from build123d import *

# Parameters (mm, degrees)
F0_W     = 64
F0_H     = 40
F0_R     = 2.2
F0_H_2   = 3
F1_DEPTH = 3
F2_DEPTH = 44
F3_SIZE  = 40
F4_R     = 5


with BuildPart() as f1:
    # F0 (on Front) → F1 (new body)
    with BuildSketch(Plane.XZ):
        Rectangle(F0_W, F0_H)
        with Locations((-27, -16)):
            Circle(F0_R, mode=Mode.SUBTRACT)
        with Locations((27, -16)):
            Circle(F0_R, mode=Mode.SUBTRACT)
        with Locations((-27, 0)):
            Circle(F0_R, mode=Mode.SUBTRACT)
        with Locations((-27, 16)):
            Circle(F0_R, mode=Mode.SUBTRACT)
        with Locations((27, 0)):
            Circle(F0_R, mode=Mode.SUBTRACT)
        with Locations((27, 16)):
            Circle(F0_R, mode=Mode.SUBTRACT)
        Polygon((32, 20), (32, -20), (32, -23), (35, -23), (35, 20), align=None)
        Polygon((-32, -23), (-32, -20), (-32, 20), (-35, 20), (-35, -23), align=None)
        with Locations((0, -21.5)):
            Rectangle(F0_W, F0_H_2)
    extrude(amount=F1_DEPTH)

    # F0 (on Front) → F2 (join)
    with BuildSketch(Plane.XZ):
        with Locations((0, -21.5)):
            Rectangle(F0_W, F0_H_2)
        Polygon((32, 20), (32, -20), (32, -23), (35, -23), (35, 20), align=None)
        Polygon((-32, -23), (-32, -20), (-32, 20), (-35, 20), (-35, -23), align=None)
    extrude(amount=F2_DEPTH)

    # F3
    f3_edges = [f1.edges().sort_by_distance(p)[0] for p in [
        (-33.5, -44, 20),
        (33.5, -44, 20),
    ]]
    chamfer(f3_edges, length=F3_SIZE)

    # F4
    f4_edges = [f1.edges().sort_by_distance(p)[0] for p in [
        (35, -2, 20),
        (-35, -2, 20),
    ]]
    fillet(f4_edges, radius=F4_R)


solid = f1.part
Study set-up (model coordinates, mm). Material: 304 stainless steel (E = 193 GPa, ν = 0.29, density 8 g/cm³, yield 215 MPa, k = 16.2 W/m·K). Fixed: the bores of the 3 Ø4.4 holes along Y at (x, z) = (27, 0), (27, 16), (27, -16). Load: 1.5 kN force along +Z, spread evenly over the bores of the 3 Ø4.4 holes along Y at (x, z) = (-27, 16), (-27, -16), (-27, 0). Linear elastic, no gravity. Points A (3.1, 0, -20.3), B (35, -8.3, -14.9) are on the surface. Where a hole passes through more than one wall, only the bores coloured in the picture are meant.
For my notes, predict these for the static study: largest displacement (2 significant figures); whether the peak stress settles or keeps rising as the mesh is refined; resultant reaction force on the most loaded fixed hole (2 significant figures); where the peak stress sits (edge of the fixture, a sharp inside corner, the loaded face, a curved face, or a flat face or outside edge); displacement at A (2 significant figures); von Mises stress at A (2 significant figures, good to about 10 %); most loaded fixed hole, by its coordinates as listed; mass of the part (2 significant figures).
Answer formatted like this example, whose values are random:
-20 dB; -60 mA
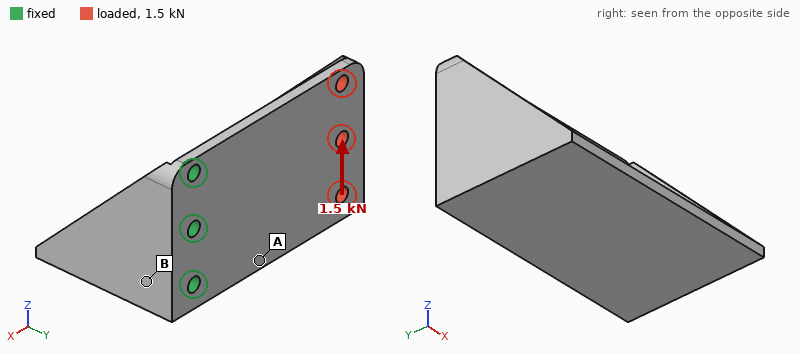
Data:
35 µm; keeps rising; 2.6 kN; edge of the fixture; 11 µm; 27 MPa; (27, -16); 180 g
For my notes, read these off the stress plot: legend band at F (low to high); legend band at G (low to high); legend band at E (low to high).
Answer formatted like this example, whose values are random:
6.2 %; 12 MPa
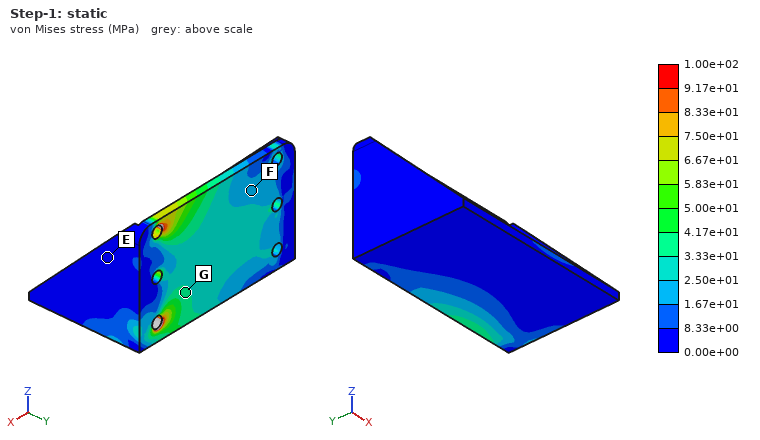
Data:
1.67e+01 to 2.50e+01 MPa; 3.33e+01 to 4.17e+01 MPa; 0.00e+00 to 8.33e+00 MPa
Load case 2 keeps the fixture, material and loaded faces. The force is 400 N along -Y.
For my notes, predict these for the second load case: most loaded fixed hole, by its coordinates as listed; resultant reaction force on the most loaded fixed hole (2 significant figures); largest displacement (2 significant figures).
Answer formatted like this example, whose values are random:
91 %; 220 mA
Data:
(27, 16); 320 N; 0.34 mm
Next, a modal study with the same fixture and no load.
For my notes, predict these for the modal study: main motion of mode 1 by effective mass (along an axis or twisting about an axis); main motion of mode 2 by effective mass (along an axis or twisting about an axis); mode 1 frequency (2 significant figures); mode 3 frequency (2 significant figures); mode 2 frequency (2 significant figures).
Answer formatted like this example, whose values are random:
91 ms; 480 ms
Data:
along Y; along Z; 740 Hz; 3100 Hz; 1100 Hz
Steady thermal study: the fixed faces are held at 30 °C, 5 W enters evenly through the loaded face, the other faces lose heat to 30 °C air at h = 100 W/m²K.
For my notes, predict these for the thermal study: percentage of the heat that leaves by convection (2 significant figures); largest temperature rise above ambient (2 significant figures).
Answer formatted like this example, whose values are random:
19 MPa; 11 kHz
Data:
97 %; 25 K
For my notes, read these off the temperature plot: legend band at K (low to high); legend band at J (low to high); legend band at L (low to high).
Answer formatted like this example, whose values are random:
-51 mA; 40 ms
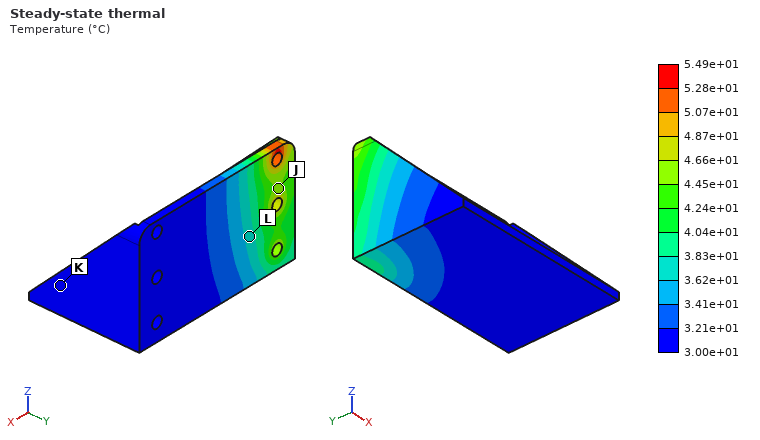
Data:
3.00e+01 to 3.21e+01 °C; 4.45e+01 to 4.66e+01 °C; 3.62e+01 to 3.83e+01 °C
